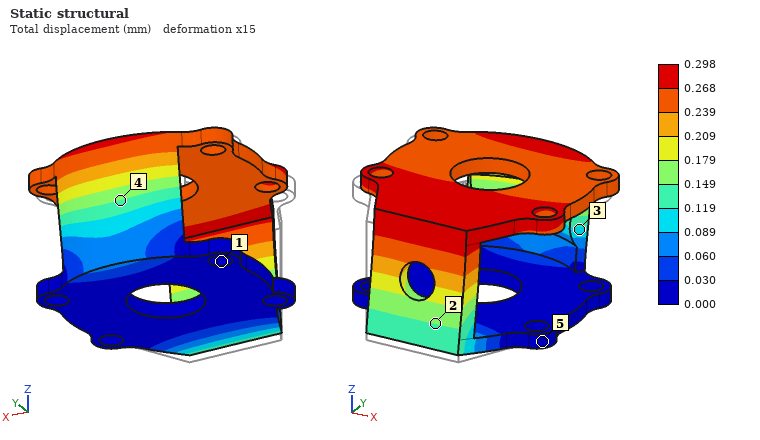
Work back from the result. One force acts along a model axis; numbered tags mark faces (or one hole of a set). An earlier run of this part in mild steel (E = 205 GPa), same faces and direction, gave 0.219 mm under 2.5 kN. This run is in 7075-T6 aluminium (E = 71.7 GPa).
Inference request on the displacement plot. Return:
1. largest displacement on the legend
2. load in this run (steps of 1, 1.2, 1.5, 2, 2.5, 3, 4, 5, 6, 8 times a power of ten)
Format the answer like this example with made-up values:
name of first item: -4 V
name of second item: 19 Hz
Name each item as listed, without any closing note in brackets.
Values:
largest displacement on the legend: 0.298 mm
load in this run: 1.2 kN
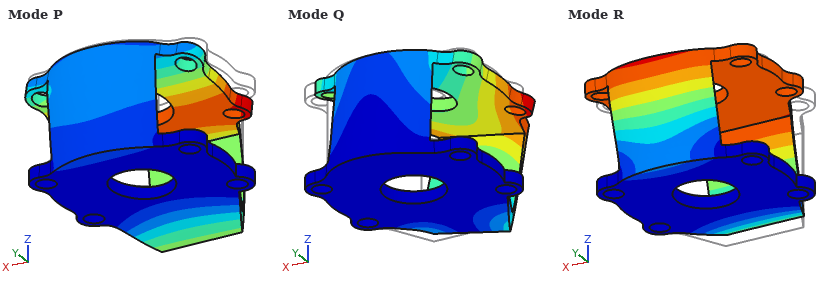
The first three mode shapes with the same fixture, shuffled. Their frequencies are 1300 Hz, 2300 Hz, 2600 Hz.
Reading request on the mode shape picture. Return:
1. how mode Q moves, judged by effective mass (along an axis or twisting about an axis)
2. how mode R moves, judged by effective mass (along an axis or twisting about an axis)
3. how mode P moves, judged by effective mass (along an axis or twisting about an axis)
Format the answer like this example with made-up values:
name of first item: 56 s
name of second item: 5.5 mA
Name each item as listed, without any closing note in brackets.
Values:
how mode Q moves, judged by effective mass: along X
how mode R moves, judged by effective mass: along Y
how mode P moves, judged by effective mass: along Z
